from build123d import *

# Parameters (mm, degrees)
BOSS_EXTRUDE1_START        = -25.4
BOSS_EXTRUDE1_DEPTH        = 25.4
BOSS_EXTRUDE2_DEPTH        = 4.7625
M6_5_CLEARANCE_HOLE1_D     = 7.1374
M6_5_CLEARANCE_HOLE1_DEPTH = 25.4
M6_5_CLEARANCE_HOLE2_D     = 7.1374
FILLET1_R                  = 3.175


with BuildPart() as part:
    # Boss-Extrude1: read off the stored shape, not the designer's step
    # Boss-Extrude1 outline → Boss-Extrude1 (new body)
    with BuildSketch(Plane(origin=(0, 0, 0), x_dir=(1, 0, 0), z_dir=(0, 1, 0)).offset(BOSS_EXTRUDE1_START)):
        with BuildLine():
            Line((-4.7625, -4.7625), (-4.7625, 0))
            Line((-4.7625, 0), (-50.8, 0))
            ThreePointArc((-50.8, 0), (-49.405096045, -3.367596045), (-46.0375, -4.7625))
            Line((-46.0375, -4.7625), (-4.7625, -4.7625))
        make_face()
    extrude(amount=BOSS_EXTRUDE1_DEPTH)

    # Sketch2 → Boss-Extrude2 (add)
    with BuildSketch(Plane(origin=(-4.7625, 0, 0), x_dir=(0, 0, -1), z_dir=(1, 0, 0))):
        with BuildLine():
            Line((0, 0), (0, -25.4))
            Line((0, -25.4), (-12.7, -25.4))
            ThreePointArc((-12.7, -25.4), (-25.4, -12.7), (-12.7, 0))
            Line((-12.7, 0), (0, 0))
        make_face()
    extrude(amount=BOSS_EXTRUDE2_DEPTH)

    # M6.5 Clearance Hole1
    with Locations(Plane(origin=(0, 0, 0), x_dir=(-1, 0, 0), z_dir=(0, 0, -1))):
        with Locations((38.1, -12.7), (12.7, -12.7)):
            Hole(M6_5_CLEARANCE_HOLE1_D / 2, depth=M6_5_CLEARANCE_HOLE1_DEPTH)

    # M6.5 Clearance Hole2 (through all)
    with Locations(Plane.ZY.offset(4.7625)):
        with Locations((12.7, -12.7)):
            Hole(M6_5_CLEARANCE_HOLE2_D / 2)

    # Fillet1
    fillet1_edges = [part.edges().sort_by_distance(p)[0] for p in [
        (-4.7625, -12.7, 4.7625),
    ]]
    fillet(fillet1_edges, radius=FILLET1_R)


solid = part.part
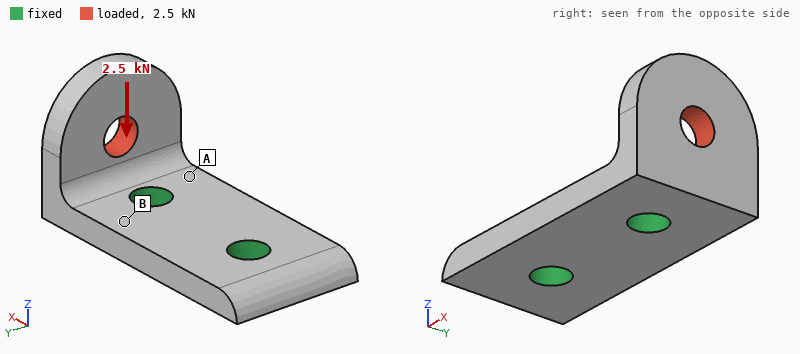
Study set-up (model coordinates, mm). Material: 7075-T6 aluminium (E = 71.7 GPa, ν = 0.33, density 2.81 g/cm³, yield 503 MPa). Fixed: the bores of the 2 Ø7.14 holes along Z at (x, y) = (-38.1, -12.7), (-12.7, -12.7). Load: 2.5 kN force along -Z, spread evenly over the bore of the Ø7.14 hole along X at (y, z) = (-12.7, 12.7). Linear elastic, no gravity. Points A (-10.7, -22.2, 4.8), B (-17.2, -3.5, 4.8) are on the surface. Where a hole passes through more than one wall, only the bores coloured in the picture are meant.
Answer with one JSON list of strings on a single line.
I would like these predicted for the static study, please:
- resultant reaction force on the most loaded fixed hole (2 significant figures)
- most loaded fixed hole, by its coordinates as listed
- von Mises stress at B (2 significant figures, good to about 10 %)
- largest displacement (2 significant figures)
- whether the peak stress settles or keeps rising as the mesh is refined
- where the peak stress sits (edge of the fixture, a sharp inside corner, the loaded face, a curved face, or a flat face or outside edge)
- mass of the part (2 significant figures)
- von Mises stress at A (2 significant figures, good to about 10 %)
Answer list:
["2.6 kN", "(-12.7, -12.7)", "32 MPa", "0.15 mm", "keeps rising", "edge of the fixture", "22 g", "81 MPa"]
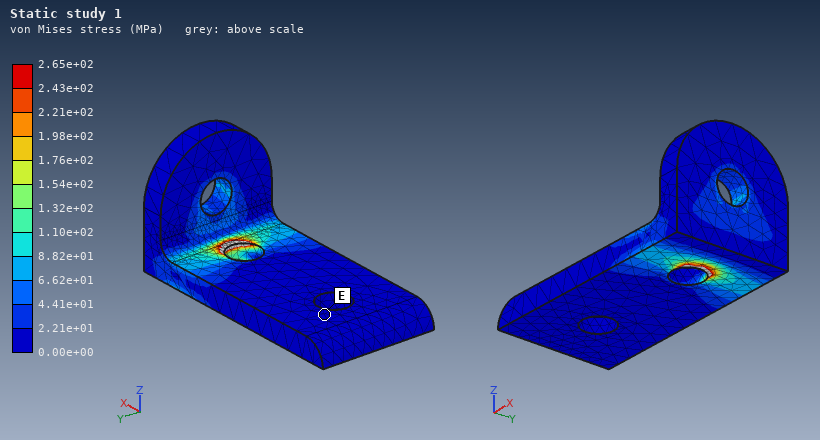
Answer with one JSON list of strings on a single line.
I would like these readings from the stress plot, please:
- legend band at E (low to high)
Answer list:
["0.00e+00 to 2.21e+01 MPa"]
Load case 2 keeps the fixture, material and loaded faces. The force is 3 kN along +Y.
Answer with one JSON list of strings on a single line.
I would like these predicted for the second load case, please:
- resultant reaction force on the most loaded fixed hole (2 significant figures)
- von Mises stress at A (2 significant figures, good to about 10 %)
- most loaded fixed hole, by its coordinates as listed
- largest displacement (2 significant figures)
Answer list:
["3.6 kN", "100 MPa", "(-12.7, -12.7)", "0.19 mm"]
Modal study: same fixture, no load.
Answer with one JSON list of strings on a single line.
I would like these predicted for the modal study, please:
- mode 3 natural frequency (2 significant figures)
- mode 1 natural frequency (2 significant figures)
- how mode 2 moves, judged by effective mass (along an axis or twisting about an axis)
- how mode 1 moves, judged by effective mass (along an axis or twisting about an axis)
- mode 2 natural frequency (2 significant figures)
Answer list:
["18 kHz", "6100 Hz", "along Y", "along X", "8500 Hz"]
